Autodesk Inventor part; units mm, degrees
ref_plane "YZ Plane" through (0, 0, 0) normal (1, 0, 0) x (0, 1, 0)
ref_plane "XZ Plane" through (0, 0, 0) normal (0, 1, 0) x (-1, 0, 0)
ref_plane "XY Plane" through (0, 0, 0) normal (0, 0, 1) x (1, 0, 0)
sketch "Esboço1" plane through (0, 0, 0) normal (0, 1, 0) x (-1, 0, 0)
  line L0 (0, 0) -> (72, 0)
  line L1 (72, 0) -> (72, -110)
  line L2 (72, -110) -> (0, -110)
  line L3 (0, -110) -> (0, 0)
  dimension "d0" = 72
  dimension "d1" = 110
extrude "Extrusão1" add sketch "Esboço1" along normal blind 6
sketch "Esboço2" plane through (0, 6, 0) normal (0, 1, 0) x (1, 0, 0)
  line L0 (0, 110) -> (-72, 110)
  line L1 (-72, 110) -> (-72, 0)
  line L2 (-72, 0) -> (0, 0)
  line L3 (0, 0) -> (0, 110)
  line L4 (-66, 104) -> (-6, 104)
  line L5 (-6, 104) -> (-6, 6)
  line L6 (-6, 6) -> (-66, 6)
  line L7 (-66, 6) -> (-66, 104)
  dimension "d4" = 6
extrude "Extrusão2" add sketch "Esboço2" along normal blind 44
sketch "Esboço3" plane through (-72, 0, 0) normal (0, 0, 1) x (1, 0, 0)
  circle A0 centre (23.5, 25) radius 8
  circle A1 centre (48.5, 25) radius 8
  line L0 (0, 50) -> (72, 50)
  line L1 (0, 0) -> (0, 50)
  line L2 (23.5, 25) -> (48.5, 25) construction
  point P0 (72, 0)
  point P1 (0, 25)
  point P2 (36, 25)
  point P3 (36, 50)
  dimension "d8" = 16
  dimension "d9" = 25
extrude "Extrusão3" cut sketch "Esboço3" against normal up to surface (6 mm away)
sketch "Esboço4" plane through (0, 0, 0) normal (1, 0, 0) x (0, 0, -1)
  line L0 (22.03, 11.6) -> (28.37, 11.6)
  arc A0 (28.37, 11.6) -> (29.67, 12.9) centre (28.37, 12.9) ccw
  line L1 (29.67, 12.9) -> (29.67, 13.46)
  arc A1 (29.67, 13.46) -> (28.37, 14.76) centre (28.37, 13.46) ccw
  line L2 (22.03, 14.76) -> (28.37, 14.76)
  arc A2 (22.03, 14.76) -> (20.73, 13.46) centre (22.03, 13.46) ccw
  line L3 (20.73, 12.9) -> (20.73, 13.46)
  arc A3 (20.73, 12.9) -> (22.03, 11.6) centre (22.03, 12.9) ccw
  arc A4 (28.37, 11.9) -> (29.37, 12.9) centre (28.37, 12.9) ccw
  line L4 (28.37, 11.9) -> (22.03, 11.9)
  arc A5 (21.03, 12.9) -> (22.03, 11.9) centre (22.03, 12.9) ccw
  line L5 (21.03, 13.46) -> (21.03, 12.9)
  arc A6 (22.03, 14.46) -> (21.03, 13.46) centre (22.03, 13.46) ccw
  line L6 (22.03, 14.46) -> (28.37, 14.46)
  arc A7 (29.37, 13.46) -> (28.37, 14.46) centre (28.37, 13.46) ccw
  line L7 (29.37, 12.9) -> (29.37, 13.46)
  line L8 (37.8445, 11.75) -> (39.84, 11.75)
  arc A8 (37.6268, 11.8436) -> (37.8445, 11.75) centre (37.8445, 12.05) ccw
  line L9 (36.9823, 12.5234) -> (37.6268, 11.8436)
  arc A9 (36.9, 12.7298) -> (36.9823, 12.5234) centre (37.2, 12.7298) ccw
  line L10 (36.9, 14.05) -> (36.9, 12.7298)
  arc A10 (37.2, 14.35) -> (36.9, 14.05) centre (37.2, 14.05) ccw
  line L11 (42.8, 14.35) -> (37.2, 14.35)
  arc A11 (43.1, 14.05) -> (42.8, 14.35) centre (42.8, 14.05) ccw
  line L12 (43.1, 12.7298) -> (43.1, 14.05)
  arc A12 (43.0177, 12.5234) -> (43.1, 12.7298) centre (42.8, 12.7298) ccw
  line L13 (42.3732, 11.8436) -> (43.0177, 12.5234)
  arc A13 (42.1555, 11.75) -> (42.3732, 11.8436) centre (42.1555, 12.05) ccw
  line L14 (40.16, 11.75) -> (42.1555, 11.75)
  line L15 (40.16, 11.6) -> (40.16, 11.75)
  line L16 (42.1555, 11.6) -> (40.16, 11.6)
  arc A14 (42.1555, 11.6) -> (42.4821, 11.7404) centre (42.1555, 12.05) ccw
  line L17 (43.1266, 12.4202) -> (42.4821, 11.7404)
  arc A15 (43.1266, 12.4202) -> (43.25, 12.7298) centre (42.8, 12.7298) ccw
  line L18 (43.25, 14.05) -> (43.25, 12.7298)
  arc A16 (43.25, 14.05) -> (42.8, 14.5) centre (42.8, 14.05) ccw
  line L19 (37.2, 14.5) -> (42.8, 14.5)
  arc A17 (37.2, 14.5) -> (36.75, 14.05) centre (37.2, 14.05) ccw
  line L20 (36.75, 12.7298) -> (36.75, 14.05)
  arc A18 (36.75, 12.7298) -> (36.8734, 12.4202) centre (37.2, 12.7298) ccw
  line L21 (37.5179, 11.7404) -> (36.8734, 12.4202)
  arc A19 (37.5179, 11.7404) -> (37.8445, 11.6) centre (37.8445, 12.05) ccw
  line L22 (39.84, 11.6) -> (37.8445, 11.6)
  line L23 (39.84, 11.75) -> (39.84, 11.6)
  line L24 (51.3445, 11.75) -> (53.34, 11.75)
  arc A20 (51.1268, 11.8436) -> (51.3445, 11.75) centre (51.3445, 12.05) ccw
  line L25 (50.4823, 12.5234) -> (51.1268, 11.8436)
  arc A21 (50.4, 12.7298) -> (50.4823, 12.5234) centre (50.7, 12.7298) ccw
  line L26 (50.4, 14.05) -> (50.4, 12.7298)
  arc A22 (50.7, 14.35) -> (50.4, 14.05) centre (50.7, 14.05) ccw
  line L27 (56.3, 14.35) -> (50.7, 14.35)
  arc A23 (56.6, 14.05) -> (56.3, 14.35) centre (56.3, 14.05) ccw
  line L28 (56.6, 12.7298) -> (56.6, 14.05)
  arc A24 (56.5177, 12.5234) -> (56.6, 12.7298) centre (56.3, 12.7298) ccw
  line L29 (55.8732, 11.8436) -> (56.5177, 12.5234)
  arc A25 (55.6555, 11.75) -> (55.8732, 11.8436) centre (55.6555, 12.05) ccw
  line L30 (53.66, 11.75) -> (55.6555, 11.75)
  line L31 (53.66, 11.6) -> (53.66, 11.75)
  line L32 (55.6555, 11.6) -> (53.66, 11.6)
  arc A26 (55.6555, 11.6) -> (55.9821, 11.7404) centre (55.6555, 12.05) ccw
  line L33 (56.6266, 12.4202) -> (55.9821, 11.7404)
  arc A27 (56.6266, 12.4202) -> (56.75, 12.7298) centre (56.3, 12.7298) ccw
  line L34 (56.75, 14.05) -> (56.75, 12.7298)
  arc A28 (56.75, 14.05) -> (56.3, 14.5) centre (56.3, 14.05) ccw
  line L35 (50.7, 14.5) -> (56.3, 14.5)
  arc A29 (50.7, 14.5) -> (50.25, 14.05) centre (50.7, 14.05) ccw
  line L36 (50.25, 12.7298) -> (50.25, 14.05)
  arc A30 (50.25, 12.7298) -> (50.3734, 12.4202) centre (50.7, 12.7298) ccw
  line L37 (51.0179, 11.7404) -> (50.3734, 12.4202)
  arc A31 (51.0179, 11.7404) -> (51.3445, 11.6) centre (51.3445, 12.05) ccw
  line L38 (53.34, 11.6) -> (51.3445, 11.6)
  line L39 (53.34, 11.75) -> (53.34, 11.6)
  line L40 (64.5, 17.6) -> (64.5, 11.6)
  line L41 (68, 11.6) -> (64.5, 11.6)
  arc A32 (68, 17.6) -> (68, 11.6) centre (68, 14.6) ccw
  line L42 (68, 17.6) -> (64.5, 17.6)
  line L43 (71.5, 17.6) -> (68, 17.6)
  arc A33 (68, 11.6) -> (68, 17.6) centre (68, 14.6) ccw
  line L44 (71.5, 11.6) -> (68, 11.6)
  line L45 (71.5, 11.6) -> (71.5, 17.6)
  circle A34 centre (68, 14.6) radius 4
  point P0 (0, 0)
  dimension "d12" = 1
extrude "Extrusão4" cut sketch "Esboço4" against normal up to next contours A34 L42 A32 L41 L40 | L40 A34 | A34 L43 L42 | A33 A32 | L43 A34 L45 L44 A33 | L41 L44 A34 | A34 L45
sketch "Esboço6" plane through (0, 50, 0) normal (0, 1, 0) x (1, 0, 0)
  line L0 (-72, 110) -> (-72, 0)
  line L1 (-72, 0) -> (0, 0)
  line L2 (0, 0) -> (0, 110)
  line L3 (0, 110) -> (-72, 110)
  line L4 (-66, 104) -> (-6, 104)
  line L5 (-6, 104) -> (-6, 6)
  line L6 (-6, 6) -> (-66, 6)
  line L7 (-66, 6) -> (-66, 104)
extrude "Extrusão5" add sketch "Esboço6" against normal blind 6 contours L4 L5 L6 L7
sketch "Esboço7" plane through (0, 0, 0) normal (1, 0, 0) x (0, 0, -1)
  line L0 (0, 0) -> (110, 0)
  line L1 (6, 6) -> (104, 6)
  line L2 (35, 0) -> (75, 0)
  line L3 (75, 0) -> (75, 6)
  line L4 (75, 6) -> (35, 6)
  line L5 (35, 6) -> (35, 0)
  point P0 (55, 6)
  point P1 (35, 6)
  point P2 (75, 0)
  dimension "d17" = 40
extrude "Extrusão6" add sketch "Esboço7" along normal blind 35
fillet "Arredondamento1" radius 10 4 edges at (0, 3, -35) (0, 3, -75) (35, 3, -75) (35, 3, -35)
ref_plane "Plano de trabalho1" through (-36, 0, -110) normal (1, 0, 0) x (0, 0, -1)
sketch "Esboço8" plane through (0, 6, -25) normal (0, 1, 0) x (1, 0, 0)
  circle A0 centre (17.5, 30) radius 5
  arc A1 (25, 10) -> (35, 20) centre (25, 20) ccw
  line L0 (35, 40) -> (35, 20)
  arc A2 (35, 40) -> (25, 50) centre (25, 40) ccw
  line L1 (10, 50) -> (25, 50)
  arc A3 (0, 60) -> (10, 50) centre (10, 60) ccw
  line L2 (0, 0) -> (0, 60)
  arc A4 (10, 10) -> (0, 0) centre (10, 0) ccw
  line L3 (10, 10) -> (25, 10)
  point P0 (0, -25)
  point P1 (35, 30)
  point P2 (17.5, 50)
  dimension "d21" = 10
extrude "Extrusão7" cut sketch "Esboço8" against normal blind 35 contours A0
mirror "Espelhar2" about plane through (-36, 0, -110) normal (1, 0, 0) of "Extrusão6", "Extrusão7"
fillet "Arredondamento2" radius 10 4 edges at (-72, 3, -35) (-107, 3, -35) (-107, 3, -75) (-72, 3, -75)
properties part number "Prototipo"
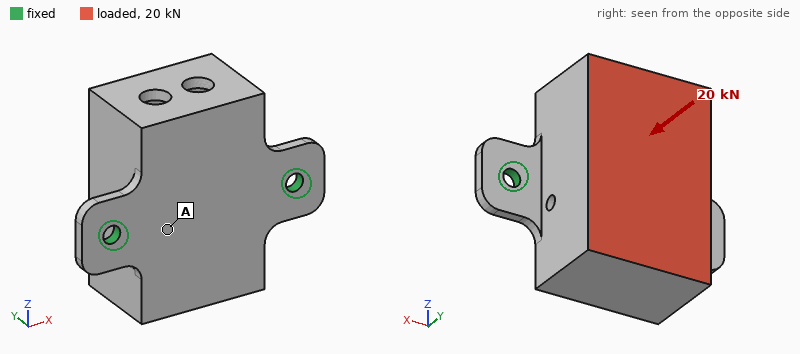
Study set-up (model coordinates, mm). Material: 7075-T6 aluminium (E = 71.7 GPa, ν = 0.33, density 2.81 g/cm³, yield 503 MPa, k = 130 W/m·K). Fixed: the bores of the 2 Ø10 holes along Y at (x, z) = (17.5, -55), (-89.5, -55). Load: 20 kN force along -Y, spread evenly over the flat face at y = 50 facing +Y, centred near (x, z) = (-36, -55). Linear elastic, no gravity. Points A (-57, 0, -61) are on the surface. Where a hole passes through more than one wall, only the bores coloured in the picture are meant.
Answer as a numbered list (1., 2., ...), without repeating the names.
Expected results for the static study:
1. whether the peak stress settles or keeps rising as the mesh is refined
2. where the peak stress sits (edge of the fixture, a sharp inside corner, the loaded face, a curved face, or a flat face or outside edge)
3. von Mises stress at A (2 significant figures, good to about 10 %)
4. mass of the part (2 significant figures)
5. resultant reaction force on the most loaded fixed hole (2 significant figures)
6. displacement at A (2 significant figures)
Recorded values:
1. keeps rising
2. edge of the fixture
3. 48 MPa
4. 520 g
5. 10 kN
6. 0.23 mm
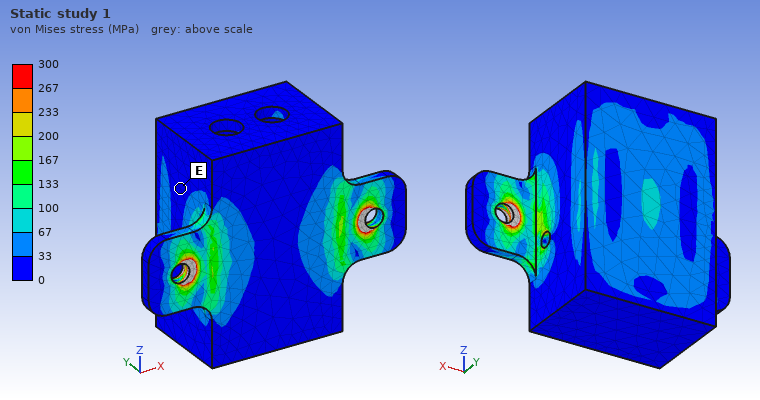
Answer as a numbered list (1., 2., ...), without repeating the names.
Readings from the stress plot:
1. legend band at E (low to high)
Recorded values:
1. 0 to 33 MPa
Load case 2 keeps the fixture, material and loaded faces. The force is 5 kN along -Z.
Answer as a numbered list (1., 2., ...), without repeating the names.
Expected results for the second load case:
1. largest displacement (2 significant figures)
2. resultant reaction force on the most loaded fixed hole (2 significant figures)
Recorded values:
1. 1.3 mm
2. 2.5 kN
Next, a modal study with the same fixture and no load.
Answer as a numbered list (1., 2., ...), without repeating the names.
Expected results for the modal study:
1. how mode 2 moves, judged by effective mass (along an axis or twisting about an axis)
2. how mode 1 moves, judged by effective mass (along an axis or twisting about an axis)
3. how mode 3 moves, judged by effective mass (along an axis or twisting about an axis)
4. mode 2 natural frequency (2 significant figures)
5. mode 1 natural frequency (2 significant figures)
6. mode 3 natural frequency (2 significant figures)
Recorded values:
1. along Y
2. along Z
3. along X
4. 2100 Hz
5. 590 Hz
6. 2300 Hz
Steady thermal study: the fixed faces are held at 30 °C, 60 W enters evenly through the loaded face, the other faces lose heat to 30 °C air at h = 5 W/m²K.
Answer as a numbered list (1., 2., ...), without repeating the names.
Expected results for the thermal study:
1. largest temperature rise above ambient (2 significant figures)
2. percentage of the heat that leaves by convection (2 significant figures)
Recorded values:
1. 35 K
2. 11 %
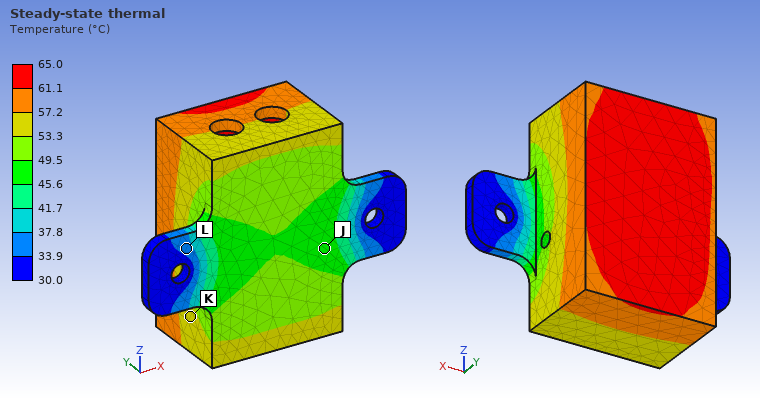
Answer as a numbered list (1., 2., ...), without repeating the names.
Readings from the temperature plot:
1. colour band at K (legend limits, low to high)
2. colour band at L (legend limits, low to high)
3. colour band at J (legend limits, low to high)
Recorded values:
1. 53.3 to 57.2 °C
2. 33.9 to 37.8 °C
3. 45.6 to 49.5 °C
